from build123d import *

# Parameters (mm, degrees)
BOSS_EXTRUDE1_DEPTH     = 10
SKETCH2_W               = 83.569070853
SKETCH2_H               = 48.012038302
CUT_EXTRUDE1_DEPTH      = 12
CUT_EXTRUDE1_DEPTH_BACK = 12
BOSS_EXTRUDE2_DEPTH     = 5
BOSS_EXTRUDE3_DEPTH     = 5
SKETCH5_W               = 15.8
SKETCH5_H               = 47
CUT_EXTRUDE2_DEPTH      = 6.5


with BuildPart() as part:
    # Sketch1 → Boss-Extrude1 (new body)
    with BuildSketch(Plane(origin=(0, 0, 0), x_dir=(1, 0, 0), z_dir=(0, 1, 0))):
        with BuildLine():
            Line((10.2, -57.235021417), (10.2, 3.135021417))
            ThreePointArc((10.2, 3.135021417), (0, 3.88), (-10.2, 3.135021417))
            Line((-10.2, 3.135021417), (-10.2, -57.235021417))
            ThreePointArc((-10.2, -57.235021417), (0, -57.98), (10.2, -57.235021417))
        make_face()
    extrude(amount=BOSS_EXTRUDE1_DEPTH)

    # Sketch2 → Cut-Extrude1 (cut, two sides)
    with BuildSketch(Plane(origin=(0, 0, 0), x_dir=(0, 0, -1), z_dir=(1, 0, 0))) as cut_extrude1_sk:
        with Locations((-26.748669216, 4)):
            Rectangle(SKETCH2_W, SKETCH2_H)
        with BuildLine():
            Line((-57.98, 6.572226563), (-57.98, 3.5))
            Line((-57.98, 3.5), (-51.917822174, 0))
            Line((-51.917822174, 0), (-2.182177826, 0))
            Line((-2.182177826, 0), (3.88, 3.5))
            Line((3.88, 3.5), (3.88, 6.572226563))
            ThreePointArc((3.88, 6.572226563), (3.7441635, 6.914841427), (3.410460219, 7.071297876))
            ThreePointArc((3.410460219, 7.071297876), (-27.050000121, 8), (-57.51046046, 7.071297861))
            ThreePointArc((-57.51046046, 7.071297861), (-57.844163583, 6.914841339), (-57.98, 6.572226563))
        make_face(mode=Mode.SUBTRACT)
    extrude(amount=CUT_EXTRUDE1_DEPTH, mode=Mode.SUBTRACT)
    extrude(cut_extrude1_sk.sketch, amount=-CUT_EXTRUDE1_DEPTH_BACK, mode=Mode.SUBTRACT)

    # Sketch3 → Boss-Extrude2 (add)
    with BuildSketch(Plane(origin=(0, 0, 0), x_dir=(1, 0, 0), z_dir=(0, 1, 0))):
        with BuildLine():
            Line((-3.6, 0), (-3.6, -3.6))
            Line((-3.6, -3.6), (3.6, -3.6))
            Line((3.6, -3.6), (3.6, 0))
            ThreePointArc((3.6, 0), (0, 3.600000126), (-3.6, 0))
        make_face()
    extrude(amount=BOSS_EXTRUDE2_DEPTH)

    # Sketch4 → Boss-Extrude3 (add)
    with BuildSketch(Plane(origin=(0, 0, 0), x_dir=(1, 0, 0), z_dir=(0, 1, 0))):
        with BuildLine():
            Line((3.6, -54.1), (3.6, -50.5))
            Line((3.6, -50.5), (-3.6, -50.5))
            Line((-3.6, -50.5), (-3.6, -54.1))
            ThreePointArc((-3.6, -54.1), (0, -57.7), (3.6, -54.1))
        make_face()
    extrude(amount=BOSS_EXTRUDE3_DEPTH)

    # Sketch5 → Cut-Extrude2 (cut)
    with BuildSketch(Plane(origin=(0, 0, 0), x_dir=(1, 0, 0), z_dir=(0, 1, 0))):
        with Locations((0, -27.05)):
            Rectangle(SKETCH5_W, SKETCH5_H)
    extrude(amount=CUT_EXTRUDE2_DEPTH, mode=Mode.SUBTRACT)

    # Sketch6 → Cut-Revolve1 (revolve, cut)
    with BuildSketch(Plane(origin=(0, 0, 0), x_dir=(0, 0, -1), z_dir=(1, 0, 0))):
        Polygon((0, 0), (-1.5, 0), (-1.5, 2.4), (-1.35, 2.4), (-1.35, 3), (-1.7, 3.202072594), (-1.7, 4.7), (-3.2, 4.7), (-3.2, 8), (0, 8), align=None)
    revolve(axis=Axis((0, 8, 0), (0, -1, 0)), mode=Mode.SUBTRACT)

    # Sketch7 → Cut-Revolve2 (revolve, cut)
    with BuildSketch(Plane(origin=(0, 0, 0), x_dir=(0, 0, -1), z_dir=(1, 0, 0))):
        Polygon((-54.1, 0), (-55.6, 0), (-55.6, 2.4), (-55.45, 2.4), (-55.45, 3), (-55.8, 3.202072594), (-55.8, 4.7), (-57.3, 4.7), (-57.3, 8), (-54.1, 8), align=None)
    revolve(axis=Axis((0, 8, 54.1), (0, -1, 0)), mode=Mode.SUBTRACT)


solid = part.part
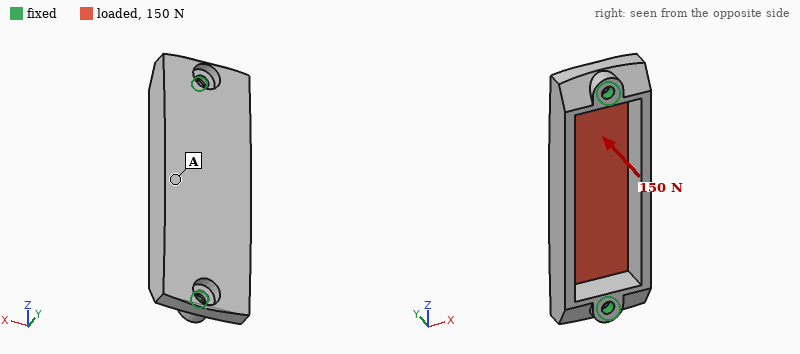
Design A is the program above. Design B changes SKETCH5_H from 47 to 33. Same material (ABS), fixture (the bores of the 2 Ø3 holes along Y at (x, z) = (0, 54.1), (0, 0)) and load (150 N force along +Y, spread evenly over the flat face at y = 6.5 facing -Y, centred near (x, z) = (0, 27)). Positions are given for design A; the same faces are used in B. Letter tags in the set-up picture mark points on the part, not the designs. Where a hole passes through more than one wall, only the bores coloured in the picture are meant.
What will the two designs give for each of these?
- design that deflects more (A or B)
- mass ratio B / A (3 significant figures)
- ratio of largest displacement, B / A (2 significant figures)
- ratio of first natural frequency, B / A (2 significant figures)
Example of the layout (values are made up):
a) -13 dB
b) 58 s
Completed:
a) A
b) 1.34
c) 0.76
d) 1.1
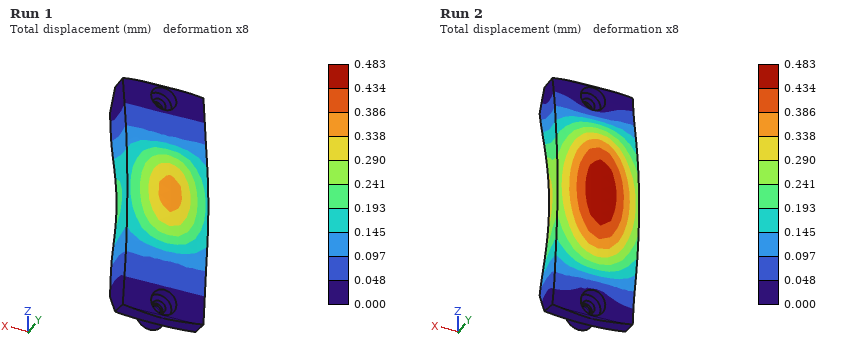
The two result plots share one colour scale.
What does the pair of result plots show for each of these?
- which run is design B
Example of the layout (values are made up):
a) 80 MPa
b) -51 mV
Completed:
a) Run 1
